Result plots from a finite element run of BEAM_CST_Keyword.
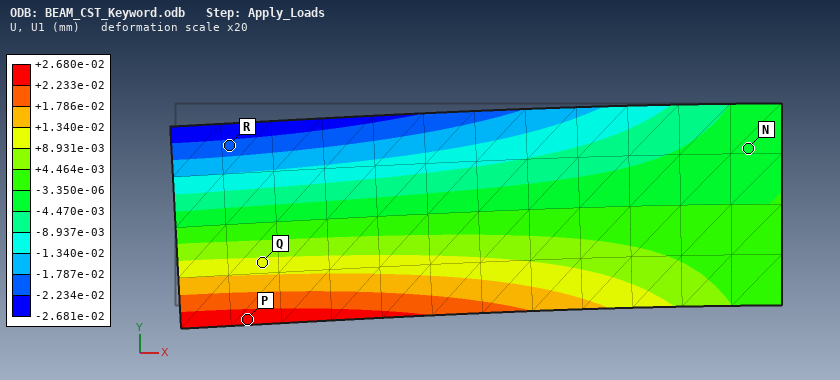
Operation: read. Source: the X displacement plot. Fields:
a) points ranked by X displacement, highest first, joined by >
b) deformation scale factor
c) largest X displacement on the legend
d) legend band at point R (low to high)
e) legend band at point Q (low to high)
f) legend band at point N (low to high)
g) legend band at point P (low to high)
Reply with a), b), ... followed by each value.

a) P > Q > N > R
b) 20
c) +2.680e-02 mm
d) -2.234e-02 to -1.787e-02 mm
e) +8.931e-03 to +1.340e-02 mm
f) -4.470e-03 to -3.350e-06 mm
g) +2.233e-02 to +2.680e-02 mm
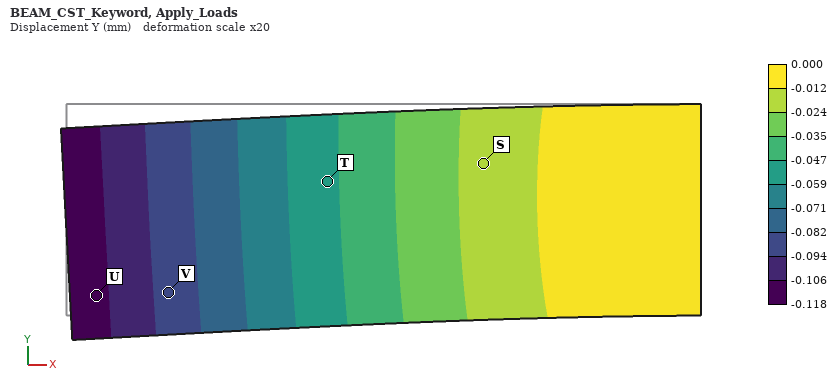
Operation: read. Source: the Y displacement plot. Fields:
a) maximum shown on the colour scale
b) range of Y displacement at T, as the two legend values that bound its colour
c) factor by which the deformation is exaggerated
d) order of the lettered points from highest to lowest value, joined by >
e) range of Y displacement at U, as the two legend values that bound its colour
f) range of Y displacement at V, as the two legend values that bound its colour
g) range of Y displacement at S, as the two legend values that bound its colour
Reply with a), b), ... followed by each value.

a) 0.000 mm
b) -0.059 to -0.047 mm
c) 20
d) S > T > V > U
e) -0.118 to -0.106 mm
f) -0.094 to -0.082 mm
g) -0.024 to -0.012 mm
